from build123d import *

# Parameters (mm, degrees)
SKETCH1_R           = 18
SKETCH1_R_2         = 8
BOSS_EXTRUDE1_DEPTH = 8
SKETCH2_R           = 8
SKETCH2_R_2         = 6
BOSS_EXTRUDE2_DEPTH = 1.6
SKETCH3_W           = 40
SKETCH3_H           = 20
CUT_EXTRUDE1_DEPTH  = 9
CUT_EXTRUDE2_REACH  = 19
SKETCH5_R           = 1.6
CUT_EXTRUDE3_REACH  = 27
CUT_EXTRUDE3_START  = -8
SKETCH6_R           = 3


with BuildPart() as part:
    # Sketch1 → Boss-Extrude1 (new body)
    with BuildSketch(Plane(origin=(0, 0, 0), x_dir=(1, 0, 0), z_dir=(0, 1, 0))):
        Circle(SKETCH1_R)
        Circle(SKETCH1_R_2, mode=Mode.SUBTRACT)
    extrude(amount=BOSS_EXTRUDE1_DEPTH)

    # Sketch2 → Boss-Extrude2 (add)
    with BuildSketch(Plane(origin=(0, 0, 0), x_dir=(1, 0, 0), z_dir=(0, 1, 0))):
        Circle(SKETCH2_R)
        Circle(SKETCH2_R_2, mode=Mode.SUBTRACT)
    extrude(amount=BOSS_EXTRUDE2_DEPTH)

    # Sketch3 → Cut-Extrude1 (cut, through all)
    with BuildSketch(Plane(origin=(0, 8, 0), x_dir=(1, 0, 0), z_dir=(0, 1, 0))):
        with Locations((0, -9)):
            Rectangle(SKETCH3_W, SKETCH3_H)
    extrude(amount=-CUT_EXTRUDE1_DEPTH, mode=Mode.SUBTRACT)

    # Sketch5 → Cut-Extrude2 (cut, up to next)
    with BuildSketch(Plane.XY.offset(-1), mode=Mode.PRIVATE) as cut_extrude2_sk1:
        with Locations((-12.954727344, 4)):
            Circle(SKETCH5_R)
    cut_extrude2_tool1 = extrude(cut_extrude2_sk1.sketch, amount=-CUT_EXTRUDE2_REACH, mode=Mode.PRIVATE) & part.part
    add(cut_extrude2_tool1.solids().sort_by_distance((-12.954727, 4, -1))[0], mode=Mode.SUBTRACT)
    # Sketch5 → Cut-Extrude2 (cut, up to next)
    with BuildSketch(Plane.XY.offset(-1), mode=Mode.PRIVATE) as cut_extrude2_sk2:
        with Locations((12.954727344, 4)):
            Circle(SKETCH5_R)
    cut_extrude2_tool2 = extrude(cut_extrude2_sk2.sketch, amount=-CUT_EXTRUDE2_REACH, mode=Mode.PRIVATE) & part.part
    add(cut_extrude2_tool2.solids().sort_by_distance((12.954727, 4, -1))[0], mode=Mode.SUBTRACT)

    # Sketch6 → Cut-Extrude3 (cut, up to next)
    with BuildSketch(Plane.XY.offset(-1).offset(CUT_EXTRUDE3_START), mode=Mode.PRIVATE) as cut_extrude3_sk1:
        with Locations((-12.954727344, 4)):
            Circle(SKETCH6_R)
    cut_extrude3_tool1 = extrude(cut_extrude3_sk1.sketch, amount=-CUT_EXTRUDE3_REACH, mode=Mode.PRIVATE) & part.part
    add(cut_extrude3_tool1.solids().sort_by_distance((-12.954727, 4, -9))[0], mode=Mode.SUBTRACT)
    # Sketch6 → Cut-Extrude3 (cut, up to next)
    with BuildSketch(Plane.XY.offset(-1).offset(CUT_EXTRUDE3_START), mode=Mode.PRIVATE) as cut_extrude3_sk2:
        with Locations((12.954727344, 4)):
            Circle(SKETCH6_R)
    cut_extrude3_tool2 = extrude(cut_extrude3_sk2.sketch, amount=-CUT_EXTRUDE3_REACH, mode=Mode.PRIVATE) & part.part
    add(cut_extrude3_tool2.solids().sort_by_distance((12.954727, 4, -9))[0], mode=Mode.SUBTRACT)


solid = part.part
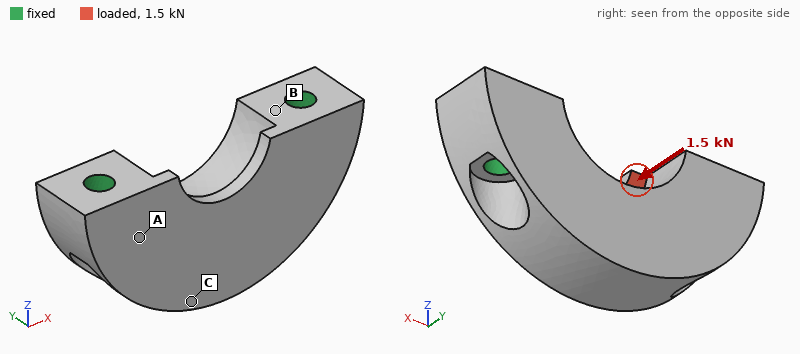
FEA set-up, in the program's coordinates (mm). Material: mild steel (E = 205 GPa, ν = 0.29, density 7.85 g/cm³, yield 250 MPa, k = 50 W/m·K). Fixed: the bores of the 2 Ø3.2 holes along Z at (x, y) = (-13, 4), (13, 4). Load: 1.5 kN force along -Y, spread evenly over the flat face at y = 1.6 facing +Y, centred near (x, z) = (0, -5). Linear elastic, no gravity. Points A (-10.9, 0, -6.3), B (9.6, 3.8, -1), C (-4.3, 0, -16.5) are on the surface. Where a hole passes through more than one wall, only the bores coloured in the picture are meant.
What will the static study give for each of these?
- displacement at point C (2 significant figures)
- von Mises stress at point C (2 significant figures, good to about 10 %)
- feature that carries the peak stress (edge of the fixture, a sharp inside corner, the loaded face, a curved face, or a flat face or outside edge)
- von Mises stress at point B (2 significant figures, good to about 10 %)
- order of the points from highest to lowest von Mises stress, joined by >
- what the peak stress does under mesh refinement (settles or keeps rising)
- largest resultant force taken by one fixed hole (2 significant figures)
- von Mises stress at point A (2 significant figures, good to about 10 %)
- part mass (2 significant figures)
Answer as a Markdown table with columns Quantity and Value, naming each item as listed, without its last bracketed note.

| Quantity | Value |
|---|---|
| displacement at point C | 1.5 µm |
| von Mises stress at point C | 13 MPa |
| feature that carries the peak stress | a sharp inside corner |
| von Mises stress at point B | 43 MPa |
| order of the points from highest to lowest von Mises stress, joined by > | B > A > C |
| what the peak stress does under mesh refinement | keeps rising |
| largest resultant force taken by one fixed hole | 760 N |
| von Mises stress at point A | 27 MPa |
| part mass | 22 g |
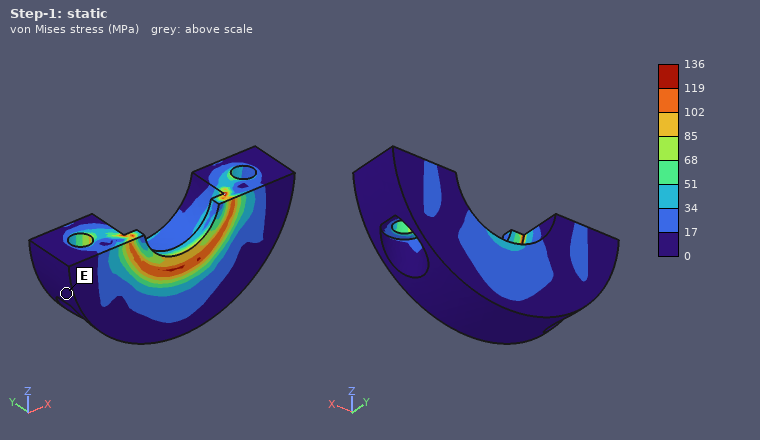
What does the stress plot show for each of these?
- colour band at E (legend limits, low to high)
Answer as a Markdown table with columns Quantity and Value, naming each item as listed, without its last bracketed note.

| Quantity | Value |
|---|---|
| colour band at E | 0 to 17 MPa |
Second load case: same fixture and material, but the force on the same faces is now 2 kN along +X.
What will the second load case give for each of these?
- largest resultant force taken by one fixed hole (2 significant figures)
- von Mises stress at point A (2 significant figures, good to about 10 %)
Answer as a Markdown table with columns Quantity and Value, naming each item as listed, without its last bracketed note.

| Quantity | Value |
|---|---|
| largest resultant force taken by one fixed hole | 1.0 kN |
| von Mises stress at point A | 23 MPa |
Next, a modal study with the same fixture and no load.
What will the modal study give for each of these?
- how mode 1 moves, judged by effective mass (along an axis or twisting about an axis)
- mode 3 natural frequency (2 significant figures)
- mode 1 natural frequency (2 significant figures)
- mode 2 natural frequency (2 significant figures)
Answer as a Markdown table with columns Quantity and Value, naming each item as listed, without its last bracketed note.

| Quantity | Value |
|---|---|
| how mode 1 moves, judged by effective mass | along Y |
| mode 3 natural frequency | 51 kHz |
| mode 1 natural frequency | 22 kHz |
| mode 2 natural frequency | 49 kHz |
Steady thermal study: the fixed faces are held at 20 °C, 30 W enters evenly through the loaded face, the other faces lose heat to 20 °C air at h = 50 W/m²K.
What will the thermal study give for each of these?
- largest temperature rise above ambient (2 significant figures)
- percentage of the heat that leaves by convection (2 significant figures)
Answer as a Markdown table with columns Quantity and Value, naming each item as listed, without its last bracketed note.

| Quantity | Value |
|---|---|
| largest temperature rise above ambient | 74 K |
| percentage of the heat that leaves by convection | 4.4 % |
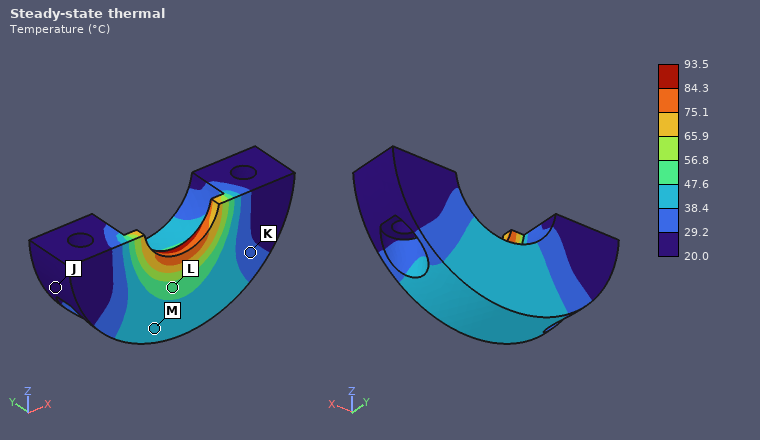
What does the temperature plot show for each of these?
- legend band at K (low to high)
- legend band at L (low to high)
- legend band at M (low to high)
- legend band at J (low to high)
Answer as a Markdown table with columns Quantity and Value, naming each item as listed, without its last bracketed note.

| Quantity | Value |
|---|---|
| legend band at K | 29.2 to 38.4 °C |
| legend band at L | 47.6 to 56.8 °C |
| legend band at M | 38.4 to 47.6 °C |
| legend band at J | 20.0 to 29.2 °C |
